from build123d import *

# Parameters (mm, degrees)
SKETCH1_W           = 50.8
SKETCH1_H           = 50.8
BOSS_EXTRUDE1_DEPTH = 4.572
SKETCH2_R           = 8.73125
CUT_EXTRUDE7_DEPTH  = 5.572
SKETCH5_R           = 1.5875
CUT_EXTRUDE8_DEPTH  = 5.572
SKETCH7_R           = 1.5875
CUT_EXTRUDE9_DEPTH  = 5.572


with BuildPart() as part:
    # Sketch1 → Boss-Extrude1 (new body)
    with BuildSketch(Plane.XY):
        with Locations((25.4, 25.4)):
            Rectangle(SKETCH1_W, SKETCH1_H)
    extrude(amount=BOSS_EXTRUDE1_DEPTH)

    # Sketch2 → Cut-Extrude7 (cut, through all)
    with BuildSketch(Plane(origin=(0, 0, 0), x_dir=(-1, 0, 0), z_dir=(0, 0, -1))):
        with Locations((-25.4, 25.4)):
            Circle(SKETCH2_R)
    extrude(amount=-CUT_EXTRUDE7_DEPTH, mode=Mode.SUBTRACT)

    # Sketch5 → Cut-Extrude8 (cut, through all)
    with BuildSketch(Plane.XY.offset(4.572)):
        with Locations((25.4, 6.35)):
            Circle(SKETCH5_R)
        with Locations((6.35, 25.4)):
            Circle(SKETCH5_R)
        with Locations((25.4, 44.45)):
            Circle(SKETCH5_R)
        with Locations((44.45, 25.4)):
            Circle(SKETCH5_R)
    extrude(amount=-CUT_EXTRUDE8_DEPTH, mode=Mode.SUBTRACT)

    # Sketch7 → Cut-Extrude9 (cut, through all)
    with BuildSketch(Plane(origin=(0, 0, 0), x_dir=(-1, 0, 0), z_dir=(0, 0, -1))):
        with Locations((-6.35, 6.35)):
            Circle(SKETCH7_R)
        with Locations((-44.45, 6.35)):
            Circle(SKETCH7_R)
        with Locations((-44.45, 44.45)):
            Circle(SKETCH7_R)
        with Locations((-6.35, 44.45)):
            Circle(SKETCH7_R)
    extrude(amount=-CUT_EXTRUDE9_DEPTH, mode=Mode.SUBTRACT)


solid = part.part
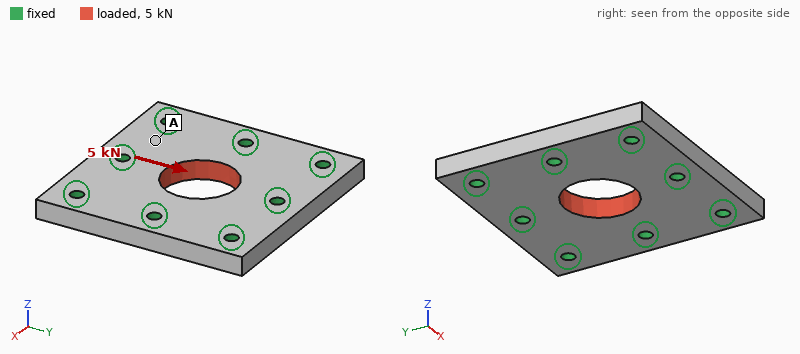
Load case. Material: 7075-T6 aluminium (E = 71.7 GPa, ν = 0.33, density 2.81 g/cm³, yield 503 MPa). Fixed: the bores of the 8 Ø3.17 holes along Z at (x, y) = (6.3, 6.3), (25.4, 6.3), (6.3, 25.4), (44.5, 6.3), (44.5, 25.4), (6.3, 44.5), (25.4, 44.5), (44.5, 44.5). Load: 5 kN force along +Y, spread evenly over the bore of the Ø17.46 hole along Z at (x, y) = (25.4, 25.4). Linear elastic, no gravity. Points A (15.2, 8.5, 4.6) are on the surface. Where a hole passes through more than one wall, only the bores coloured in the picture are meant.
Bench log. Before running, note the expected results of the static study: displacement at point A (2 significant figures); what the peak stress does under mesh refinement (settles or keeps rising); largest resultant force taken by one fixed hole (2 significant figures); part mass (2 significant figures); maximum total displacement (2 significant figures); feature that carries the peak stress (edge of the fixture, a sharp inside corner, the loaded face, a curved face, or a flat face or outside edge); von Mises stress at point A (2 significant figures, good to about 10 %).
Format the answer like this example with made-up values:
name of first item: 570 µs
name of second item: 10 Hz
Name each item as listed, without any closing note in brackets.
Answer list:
displacement at point A: 1.6 µm
what the peak stress does under mesh refinement: keeps rising
largest resultant force taken by one fixed hole: 1.2 kN
part mass: 29 g
maximum total displacement: 4.4 µm
feature that carries the peak stress: edge of the fixture
von Mises stress at point A: 8.2 MPa
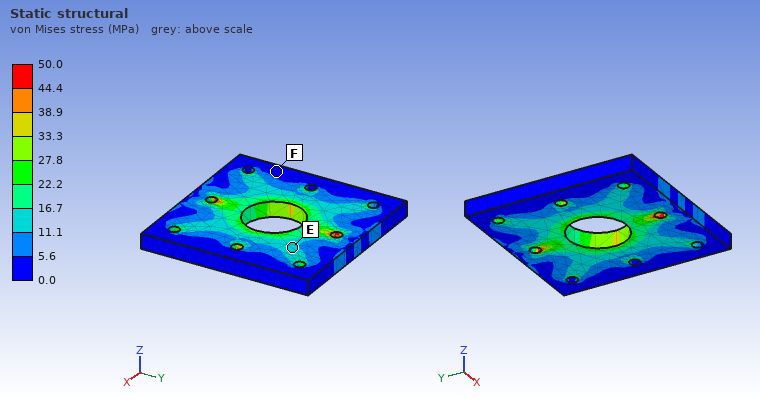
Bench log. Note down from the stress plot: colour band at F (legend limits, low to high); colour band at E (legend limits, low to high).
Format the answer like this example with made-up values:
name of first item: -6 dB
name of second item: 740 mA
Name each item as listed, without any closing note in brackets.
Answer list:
colour band at F: 0.0 to 5.6 MPa
colour band at E: 11.1 to 16.7 MPa
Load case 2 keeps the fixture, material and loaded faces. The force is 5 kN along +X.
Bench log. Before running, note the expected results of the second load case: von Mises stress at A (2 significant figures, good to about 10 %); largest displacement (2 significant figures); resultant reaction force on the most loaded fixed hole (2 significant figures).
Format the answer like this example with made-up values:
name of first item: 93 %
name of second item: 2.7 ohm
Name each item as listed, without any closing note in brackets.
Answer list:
von Mises stress at A: 8.5 MPa
largest displacement: 4.4 µm
resultant reaction force on the most loaded fixed hole: 1.2 kN
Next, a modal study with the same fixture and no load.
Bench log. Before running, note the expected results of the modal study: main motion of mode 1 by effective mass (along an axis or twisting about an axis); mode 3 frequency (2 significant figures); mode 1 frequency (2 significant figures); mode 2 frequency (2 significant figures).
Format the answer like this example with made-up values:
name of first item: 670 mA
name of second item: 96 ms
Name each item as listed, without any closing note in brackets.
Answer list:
main motion of mode 1 by effective mass: along Z
mode 3 frequency: 35 kHz
mode 1 frequency: 28 kHz
mode 2 frequency: 35 kHz
